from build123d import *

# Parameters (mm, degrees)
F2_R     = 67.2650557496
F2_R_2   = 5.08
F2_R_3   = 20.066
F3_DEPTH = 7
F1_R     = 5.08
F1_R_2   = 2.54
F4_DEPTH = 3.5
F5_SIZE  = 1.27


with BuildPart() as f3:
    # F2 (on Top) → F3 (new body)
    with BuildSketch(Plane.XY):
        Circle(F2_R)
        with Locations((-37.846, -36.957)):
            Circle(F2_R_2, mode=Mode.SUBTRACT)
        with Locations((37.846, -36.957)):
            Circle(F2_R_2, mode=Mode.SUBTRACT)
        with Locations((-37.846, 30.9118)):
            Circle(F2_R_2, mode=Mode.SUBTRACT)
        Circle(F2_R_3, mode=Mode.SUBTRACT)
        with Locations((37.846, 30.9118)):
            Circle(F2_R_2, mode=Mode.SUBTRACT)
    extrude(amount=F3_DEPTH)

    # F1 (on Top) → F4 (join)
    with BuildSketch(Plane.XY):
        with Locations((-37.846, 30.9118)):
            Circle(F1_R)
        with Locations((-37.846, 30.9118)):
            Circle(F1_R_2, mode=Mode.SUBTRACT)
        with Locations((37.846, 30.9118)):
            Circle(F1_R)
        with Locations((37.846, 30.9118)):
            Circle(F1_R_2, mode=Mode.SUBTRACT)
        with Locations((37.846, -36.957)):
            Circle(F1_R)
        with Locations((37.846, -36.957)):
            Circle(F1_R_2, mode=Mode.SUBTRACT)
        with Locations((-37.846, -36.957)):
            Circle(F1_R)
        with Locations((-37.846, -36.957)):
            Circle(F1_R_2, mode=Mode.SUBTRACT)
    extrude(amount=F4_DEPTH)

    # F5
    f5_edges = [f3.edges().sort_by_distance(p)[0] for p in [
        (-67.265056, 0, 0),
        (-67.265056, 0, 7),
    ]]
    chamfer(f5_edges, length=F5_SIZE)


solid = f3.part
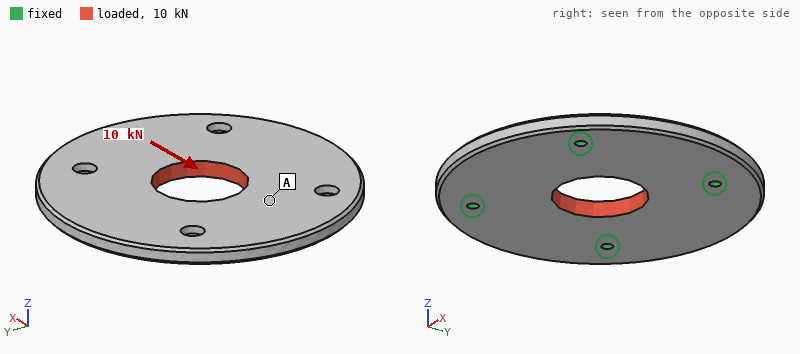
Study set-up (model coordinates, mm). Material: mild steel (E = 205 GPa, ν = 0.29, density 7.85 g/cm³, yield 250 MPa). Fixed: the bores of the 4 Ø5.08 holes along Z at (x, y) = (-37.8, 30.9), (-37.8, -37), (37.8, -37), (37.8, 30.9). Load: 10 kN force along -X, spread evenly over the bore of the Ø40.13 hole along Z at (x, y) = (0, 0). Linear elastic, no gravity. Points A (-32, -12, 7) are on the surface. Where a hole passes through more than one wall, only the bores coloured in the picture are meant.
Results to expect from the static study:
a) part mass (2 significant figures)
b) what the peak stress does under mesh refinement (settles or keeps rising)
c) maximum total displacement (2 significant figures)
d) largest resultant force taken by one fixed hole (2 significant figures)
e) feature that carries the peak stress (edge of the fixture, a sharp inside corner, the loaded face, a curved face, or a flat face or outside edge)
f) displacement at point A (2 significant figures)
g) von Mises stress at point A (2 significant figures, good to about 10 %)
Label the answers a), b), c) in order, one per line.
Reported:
a) 700 g
b) keeps rising
c) 4.8 µm
d) 2.7 kN
e) edge of the fixture
f) 3.3 µm
g) 7.6 MPa
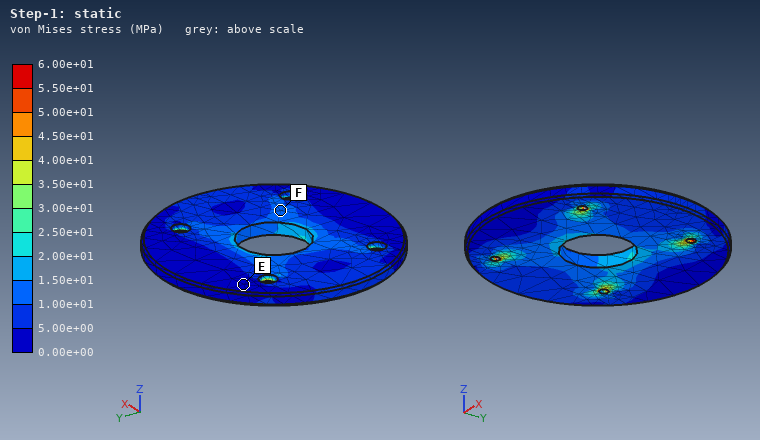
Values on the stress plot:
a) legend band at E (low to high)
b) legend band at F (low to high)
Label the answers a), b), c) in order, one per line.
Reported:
a) 0.00e+00 to 5.00e+00 MPa
b) 1.00e+01 to 1.50e+01 MPa
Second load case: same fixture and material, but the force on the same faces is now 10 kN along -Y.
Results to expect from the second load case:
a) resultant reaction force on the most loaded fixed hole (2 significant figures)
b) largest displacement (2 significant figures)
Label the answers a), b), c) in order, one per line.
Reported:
a) 2.6 kN
b) 6.1 µm
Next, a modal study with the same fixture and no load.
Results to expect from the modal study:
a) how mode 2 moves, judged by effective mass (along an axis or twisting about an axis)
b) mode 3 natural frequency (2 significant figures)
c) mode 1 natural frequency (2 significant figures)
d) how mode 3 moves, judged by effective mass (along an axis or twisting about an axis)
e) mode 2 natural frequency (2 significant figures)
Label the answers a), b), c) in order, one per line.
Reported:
a) twisting about X
b) 4100 Hz
c) 2800 Hz
d) twisting about Y
e) 3400 Hz
